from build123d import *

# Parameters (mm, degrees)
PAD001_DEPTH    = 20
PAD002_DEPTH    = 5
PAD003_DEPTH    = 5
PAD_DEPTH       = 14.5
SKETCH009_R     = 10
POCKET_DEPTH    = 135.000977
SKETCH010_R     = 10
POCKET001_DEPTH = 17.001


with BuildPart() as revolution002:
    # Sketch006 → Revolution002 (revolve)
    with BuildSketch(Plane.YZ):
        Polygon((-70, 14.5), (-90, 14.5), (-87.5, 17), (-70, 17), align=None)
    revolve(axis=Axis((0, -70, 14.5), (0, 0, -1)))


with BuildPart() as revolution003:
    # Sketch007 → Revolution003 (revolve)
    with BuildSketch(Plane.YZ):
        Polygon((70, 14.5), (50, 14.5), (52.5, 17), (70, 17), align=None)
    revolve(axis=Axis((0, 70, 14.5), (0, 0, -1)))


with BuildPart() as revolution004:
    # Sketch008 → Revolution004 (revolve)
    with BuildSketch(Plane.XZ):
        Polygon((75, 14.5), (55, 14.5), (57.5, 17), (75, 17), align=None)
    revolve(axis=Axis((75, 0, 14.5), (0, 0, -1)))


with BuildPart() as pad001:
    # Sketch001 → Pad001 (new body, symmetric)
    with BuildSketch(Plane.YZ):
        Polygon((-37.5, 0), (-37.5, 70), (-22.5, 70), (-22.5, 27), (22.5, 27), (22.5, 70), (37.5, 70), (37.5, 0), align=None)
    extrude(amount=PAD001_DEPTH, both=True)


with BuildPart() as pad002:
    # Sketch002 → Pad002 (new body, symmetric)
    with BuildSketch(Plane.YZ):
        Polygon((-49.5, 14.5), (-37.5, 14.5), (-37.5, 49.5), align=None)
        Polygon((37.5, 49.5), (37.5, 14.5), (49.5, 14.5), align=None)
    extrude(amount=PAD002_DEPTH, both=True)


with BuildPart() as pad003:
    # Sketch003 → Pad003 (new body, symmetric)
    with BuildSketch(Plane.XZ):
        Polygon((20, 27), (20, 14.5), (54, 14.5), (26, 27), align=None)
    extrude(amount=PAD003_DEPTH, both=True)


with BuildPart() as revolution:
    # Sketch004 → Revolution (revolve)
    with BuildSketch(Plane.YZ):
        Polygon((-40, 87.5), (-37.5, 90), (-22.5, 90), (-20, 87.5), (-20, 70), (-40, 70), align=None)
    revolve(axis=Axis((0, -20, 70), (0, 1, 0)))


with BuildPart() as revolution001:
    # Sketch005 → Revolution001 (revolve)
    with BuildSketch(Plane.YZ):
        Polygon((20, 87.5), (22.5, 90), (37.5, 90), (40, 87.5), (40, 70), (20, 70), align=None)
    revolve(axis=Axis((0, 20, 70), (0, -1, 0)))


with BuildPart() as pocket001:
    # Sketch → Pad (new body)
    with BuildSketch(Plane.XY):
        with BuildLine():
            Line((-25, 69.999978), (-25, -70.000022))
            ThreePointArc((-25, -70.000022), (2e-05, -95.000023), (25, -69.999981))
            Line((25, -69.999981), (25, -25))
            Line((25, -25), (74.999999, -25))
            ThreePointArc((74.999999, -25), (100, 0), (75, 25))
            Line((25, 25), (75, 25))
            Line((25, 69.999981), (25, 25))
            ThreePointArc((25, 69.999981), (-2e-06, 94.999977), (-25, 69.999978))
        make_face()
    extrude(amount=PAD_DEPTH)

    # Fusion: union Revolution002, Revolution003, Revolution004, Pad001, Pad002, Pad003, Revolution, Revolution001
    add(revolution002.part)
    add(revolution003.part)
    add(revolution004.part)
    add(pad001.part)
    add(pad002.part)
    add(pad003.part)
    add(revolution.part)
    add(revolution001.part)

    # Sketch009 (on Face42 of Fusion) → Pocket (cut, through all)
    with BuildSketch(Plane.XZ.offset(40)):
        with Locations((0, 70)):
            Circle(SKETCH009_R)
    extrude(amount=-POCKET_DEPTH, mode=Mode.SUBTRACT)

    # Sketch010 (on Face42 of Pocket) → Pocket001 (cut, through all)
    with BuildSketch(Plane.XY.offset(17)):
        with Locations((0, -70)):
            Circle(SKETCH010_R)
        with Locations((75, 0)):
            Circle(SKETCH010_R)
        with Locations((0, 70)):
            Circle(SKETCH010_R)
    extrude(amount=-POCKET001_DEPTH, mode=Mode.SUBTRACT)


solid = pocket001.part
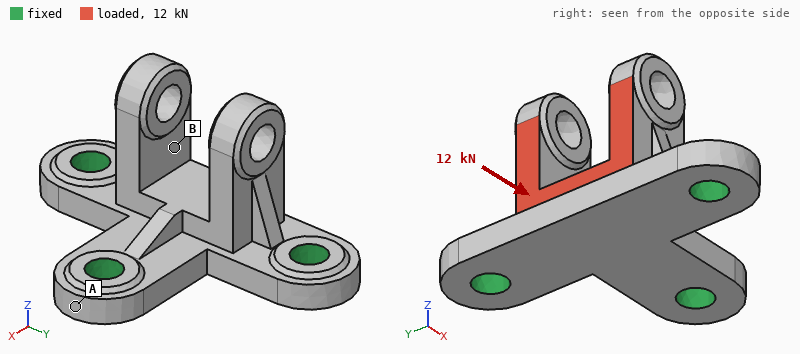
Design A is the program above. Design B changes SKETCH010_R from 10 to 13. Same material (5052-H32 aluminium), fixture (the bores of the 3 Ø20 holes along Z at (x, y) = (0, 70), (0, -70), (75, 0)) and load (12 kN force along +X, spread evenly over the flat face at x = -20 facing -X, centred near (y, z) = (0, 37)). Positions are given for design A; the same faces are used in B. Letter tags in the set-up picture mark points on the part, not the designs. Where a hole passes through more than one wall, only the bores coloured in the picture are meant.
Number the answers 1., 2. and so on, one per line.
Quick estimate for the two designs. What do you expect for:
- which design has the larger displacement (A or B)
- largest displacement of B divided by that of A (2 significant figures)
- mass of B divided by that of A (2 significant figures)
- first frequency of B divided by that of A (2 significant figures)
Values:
1. A
2. 0.91
3. 0.96
4. 1.0
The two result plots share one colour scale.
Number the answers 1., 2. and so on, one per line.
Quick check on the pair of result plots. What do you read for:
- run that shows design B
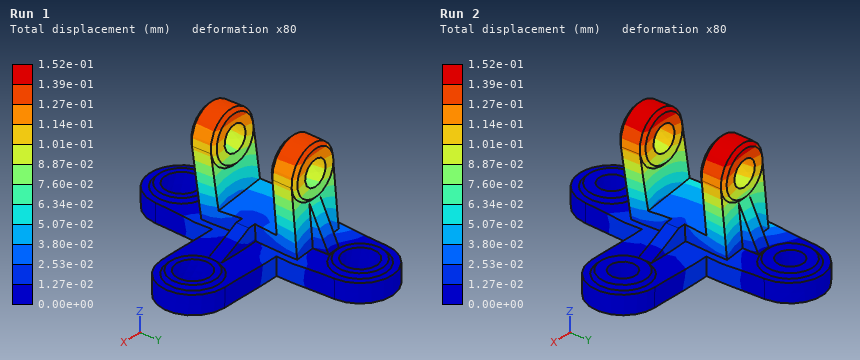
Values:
1. Run 1
